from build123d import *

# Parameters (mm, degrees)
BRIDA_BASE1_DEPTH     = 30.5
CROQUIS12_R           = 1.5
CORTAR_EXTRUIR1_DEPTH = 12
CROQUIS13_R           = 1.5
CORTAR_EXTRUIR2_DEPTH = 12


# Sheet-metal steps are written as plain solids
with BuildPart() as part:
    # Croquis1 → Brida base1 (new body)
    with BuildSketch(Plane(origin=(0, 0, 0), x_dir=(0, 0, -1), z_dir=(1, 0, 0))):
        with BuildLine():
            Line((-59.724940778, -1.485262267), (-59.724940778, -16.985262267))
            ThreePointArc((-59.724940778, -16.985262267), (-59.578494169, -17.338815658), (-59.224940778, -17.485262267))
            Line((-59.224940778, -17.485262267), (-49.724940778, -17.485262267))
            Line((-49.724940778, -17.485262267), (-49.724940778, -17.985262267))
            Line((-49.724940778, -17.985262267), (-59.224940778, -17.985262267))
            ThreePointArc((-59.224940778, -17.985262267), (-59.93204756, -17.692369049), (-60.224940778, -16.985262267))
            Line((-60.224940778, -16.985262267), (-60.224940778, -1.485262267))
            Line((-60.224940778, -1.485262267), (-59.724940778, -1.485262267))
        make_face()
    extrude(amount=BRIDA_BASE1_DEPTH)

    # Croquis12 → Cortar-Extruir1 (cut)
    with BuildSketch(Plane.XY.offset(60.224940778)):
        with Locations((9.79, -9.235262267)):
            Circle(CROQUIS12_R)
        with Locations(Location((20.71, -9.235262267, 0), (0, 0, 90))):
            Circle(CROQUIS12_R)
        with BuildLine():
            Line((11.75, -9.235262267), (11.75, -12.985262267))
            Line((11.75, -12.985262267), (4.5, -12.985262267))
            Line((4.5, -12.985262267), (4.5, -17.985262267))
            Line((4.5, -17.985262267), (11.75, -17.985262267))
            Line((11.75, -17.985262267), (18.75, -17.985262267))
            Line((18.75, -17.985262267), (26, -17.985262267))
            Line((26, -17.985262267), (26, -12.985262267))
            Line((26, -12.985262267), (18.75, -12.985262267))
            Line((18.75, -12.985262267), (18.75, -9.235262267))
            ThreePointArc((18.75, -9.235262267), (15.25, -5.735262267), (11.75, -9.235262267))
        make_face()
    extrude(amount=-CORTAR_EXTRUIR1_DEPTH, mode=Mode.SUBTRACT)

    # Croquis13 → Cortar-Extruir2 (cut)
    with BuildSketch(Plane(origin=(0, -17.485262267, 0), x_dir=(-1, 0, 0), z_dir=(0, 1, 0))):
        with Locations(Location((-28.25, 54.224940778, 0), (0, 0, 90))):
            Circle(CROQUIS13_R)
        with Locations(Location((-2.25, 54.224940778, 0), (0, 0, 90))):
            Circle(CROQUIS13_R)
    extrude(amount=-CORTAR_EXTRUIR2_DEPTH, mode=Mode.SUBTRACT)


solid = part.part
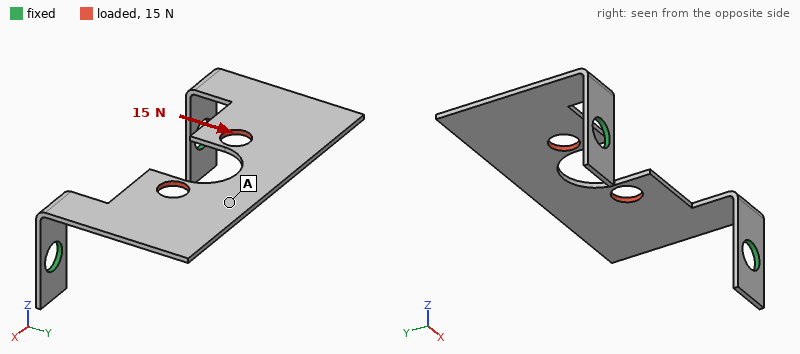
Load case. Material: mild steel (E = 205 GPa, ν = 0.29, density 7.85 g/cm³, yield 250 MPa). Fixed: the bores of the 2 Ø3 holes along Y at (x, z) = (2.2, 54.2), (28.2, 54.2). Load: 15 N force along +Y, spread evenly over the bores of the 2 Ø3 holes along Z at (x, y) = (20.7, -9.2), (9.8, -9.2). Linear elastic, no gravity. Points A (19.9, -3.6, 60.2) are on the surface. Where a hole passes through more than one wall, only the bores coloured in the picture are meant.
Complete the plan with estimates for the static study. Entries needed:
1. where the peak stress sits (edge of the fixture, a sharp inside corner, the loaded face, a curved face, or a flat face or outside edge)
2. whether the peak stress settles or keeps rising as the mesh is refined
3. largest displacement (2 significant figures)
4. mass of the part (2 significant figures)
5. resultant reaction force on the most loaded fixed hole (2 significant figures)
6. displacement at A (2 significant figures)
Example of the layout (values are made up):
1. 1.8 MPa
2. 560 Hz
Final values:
1. edge of the fixture
2. keeps rising
3. 0.12 mm
4. 1.6 g
5. 8.2 N
6. 0.11 mm
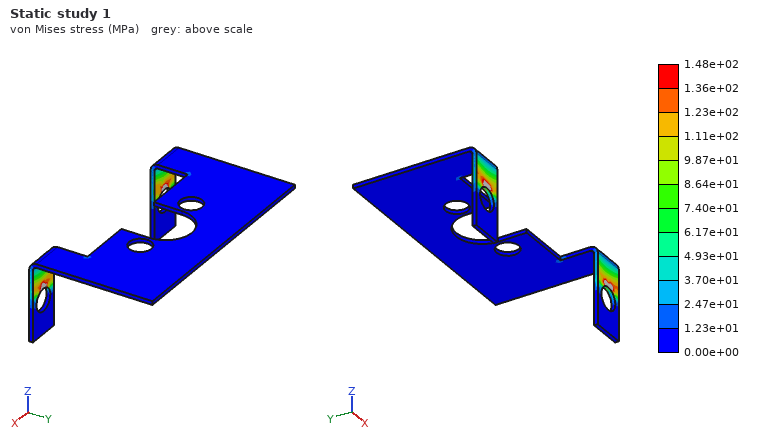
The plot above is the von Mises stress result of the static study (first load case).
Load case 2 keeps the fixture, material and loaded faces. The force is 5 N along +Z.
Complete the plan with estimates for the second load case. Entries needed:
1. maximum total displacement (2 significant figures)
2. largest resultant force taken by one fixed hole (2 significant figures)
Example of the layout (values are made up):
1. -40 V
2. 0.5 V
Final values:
1. 0.31 mm
2. 2.5 N
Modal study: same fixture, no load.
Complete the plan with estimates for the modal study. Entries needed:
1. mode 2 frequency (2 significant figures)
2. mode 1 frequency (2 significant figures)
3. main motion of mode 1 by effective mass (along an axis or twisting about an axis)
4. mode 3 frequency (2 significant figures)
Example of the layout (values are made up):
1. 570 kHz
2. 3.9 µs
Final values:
1. 1600 Hz
2. 630 Hz
3. along Z
4. 3500 Hz
